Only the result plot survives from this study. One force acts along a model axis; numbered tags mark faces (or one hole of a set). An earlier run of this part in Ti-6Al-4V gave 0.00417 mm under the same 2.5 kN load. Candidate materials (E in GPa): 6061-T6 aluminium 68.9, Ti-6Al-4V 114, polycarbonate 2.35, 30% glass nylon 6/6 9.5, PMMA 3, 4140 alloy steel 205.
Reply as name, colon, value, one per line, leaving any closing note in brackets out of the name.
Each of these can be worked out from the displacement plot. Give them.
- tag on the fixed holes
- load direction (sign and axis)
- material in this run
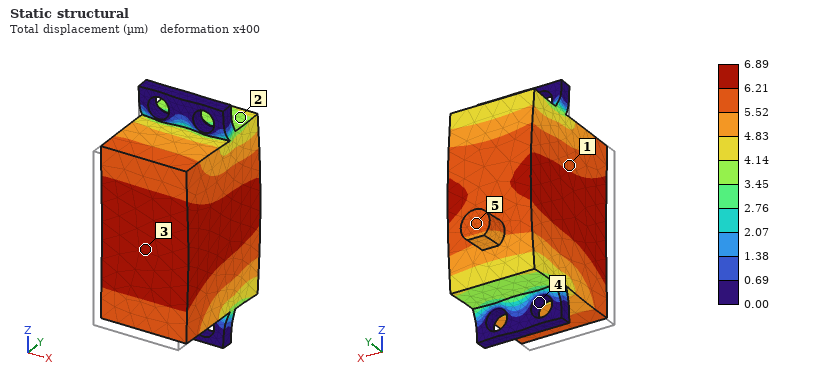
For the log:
tag on the fixed holes: 4
load direction: +Y
material in this run: 6061-T6 aluminium
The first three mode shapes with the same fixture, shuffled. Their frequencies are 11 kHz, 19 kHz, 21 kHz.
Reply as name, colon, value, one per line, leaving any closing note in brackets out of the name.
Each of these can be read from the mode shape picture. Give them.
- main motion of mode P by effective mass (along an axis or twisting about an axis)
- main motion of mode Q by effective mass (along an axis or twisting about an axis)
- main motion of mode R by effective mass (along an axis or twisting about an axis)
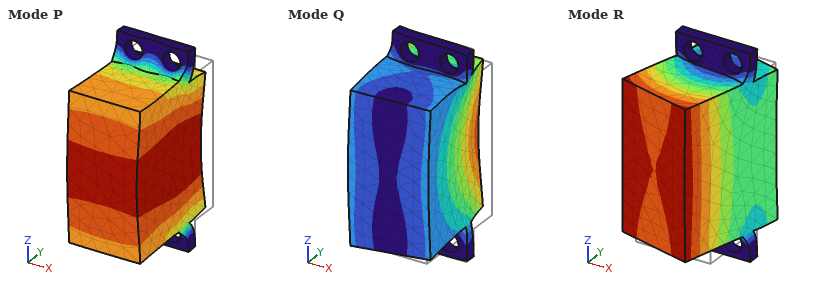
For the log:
main motion of mode P by effective mass: along Y
main motion of mode Q by effective mass: along X
main motion of mode R by effective mass: along X
